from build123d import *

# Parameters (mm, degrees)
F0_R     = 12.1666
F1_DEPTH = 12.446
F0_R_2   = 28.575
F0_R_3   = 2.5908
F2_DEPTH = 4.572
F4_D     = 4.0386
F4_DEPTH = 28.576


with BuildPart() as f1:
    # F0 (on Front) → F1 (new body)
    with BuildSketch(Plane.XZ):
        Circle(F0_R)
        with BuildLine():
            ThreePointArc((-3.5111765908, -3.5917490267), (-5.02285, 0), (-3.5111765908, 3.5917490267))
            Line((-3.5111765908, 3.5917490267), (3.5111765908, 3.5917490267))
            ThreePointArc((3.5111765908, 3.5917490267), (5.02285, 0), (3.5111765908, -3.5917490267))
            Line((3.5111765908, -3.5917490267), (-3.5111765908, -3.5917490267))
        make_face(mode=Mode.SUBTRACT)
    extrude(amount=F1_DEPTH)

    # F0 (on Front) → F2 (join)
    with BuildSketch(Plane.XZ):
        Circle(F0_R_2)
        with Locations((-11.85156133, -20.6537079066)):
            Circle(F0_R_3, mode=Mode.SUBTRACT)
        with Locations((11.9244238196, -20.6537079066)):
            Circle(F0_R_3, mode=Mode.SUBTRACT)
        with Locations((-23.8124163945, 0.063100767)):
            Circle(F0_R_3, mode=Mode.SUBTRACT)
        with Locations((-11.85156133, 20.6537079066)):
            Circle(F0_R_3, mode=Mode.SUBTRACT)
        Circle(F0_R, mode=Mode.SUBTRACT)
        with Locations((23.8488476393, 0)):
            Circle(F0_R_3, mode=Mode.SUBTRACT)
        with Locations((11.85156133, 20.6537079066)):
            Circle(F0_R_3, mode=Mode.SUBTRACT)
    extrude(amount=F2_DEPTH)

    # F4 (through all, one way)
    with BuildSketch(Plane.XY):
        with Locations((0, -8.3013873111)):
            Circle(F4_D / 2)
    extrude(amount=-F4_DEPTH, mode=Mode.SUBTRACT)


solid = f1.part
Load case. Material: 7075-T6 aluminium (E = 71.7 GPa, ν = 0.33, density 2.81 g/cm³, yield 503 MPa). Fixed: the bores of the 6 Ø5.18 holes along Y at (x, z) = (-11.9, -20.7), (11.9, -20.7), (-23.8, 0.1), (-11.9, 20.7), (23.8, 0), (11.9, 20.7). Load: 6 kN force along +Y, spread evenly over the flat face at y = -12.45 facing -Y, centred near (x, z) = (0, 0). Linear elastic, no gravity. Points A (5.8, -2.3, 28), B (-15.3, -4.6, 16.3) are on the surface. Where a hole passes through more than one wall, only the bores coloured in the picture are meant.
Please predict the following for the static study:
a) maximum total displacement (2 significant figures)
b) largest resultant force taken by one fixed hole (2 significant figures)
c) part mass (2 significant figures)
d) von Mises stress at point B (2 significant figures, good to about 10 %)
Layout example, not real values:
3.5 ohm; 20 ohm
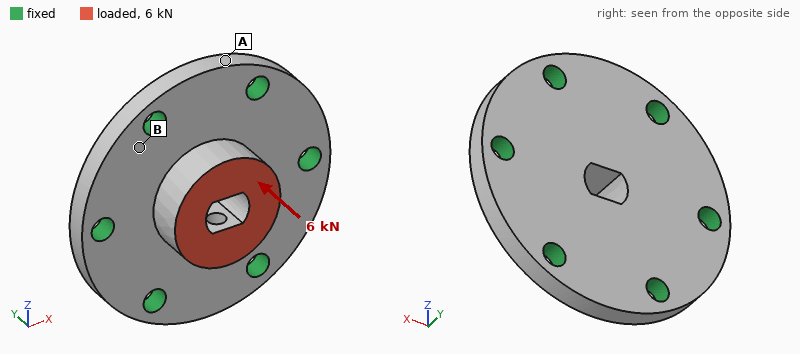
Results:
33 µm; 1.1 kN; 39 g; 34 MPa
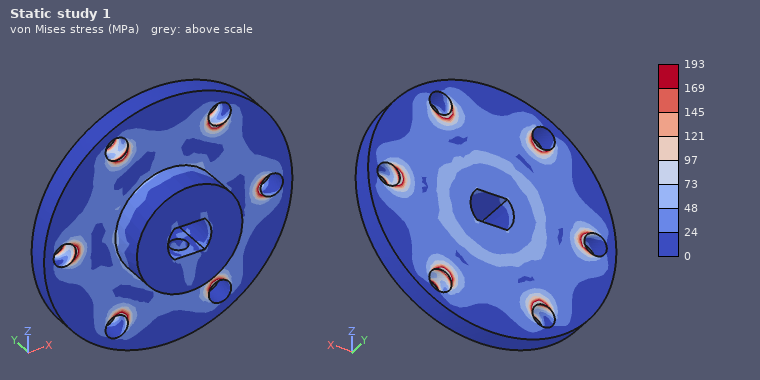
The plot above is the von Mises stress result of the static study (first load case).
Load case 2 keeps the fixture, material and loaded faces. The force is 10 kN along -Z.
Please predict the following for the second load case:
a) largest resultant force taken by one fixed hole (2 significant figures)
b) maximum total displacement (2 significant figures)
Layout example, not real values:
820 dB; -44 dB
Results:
2.7 kN; 66 µm
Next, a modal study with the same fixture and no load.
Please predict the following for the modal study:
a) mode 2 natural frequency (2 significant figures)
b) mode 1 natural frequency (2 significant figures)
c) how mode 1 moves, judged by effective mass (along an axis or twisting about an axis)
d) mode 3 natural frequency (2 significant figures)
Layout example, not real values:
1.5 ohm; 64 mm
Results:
25 kHz; 17 kHz; along Y; 25 kHz
